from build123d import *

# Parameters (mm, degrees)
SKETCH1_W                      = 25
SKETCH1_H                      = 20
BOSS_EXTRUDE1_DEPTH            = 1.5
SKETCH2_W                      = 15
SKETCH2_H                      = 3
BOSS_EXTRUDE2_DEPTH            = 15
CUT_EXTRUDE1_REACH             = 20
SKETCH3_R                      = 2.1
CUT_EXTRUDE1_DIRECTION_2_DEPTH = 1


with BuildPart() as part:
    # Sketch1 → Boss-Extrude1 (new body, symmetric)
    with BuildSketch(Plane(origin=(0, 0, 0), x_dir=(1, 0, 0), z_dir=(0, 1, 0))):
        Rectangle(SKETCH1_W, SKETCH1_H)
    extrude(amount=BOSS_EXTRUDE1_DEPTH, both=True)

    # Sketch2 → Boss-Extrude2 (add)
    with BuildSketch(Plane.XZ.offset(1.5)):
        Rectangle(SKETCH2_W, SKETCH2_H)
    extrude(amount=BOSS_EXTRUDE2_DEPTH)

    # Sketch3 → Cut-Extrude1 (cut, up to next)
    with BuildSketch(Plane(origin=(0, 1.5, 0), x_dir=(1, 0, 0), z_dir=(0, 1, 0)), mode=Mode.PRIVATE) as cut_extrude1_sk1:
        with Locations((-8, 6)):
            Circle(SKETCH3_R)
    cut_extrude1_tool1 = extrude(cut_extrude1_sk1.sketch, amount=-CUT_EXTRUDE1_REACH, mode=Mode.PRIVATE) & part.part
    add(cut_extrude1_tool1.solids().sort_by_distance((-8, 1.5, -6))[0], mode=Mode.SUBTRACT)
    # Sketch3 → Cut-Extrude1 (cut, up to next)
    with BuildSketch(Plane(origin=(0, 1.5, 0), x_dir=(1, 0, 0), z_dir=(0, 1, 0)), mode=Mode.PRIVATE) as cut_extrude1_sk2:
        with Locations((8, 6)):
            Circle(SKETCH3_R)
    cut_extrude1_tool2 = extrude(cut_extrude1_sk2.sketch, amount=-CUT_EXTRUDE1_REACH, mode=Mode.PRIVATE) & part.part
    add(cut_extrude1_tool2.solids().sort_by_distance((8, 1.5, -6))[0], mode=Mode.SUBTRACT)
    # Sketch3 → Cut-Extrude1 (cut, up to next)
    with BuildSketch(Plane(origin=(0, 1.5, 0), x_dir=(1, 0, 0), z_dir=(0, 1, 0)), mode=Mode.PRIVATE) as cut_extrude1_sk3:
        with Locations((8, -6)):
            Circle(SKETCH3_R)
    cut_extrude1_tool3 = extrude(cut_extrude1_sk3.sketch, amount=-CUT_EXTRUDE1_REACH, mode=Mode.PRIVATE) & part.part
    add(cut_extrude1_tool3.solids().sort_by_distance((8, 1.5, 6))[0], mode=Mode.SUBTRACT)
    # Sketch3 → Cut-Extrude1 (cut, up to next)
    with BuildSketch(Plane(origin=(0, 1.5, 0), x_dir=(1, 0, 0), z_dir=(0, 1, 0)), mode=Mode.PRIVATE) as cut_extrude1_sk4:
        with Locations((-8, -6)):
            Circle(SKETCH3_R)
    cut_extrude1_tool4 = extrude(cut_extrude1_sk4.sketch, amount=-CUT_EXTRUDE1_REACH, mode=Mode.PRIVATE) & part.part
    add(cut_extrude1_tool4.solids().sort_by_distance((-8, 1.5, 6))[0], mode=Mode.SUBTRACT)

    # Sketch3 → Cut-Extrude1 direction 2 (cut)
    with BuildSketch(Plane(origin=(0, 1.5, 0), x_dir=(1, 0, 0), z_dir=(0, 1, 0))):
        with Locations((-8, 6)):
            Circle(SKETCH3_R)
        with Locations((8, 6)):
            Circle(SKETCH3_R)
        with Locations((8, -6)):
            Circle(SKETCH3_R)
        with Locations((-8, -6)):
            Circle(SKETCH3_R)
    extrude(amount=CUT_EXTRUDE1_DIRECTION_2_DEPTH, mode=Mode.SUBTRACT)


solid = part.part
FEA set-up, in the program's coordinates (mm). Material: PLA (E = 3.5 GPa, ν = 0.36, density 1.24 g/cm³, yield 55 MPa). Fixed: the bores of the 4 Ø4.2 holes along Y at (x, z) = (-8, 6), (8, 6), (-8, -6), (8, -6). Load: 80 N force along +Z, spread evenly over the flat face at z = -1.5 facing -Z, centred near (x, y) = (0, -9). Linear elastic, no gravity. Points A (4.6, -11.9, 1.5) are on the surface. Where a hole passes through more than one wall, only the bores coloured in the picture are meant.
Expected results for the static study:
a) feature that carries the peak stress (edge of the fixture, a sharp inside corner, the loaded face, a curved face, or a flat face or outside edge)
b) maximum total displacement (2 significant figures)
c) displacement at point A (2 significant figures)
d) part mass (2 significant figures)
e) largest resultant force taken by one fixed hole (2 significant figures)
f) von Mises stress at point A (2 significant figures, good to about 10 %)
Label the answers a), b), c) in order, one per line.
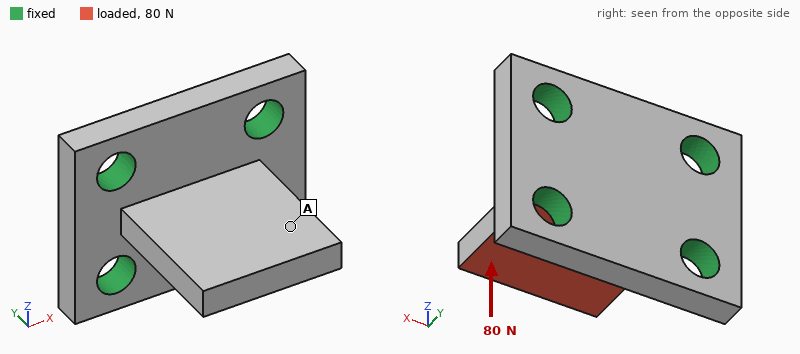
a) the loaded face
b) 0.39 mm
c) 0.25 mm
d) 2.5 g
e) 47 N
f) 2.9 MPa
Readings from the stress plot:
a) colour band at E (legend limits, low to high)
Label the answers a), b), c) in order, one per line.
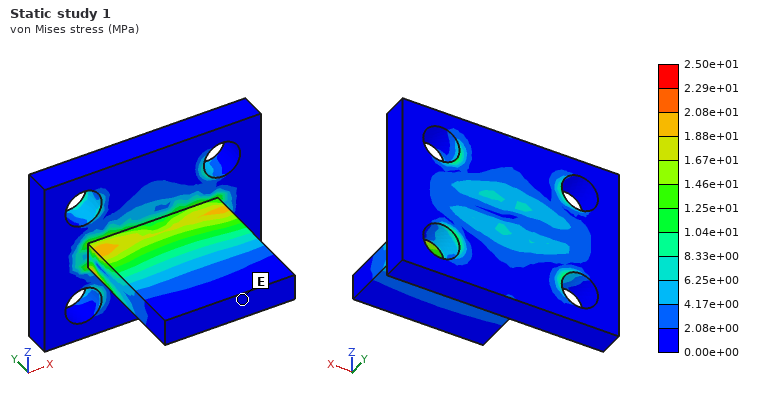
a) 0.00e+00 to 2.08e+00 MPa
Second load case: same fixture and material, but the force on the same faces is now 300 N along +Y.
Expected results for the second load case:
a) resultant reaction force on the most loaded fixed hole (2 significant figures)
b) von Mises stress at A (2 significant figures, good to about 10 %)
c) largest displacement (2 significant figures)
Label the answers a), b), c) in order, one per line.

a) 100 N
b) 4.2 MPa
c) 0.36 mm
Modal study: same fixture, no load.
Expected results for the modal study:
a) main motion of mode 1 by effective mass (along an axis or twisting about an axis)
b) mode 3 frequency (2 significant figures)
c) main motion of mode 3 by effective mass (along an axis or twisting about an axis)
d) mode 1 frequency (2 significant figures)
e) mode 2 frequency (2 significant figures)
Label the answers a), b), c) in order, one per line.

a) along Z
b) 8700 Hz
c) along X
d) 3100 Hz
e) 7300 Hz
